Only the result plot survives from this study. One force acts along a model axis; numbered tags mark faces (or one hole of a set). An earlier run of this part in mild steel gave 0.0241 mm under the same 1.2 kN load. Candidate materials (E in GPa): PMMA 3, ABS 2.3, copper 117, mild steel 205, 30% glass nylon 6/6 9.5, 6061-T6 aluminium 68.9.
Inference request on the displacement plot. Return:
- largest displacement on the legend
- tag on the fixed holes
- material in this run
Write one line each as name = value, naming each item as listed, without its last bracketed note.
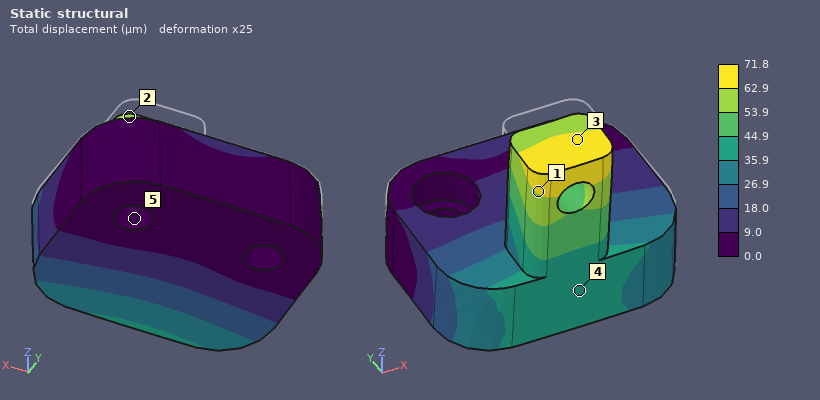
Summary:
largest displacement on the legend = 71.8 µm
tag on the fixed holes = 5
material in this run = 6061-T6 aluminium
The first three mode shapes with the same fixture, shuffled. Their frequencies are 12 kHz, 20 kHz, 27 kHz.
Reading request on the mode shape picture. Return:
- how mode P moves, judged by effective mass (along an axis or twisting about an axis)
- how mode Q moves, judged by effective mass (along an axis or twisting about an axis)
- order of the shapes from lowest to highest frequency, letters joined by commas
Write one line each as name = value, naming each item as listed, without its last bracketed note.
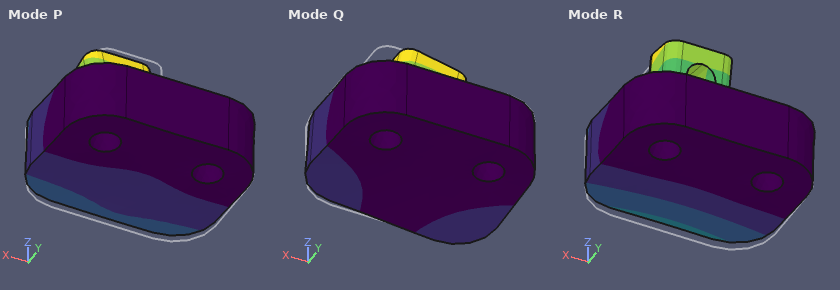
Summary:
how mode P moves, judged by effective mass = along Z
how mode Q moves, judged by effective mass = along X
order of the shapes from lowest to highest frequency, letters joined by commas = R, Q, P
